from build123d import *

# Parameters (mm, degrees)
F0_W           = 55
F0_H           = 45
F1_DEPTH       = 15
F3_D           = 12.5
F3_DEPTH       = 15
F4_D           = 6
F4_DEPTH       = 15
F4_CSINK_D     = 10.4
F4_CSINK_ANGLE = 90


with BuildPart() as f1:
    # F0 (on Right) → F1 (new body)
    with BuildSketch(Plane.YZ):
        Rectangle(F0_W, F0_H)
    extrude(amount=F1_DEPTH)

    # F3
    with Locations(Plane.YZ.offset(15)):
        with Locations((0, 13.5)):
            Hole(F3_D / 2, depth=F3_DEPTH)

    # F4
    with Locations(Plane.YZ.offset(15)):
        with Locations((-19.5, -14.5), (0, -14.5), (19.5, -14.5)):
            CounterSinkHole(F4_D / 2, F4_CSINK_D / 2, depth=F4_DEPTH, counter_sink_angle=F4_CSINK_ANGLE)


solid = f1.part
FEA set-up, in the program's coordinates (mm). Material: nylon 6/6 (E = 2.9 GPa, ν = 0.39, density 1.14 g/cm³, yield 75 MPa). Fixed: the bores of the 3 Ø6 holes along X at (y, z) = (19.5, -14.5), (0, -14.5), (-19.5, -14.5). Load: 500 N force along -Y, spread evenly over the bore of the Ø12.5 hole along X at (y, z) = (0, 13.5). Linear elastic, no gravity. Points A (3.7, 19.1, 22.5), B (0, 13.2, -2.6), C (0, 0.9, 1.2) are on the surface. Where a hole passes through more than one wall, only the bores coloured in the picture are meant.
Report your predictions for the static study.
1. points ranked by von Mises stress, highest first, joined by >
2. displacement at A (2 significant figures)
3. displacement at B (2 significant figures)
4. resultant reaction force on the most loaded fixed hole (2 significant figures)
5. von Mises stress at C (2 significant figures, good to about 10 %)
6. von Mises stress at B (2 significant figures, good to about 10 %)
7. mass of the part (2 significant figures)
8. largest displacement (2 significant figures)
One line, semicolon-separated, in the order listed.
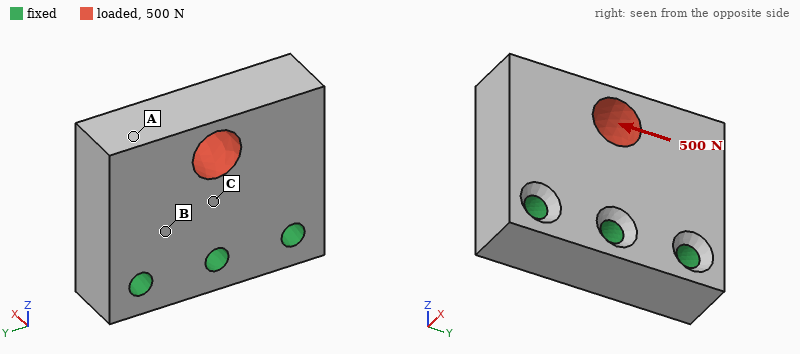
C > B > A; 36 µm; 8.8 µm; 350 N; 2.2 MPa; 1.4 MPa; 39 g; 38 µm
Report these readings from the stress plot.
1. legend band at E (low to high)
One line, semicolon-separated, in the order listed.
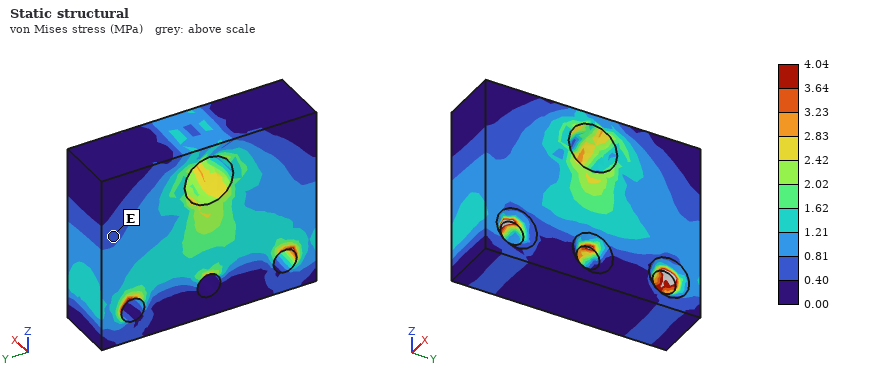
0.40 to 0.81 MPa
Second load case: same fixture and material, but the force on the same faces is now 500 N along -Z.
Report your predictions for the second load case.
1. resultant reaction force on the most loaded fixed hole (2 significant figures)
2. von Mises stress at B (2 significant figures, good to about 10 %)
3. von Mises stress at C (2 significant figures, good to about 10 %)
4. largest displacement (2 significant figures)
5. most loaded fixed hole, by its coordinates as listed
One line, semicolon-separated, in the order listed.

200 N; 0.80 MPa; 0.98 MPa; 25 µm; (0, -14.5)
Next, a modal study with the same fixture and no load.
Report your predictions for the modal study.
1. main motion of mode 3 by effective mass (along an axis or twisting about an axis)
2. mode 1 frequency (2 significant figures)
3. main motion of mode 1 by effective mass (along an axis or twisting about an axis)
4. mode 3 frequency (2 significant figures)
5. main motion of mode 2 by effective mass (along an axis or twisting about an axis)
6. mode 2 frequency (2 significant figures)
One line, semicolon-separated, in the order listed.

along Y; 2600 Hz; along X; 5000 Hz; twisting about Z; 3700 Hz
